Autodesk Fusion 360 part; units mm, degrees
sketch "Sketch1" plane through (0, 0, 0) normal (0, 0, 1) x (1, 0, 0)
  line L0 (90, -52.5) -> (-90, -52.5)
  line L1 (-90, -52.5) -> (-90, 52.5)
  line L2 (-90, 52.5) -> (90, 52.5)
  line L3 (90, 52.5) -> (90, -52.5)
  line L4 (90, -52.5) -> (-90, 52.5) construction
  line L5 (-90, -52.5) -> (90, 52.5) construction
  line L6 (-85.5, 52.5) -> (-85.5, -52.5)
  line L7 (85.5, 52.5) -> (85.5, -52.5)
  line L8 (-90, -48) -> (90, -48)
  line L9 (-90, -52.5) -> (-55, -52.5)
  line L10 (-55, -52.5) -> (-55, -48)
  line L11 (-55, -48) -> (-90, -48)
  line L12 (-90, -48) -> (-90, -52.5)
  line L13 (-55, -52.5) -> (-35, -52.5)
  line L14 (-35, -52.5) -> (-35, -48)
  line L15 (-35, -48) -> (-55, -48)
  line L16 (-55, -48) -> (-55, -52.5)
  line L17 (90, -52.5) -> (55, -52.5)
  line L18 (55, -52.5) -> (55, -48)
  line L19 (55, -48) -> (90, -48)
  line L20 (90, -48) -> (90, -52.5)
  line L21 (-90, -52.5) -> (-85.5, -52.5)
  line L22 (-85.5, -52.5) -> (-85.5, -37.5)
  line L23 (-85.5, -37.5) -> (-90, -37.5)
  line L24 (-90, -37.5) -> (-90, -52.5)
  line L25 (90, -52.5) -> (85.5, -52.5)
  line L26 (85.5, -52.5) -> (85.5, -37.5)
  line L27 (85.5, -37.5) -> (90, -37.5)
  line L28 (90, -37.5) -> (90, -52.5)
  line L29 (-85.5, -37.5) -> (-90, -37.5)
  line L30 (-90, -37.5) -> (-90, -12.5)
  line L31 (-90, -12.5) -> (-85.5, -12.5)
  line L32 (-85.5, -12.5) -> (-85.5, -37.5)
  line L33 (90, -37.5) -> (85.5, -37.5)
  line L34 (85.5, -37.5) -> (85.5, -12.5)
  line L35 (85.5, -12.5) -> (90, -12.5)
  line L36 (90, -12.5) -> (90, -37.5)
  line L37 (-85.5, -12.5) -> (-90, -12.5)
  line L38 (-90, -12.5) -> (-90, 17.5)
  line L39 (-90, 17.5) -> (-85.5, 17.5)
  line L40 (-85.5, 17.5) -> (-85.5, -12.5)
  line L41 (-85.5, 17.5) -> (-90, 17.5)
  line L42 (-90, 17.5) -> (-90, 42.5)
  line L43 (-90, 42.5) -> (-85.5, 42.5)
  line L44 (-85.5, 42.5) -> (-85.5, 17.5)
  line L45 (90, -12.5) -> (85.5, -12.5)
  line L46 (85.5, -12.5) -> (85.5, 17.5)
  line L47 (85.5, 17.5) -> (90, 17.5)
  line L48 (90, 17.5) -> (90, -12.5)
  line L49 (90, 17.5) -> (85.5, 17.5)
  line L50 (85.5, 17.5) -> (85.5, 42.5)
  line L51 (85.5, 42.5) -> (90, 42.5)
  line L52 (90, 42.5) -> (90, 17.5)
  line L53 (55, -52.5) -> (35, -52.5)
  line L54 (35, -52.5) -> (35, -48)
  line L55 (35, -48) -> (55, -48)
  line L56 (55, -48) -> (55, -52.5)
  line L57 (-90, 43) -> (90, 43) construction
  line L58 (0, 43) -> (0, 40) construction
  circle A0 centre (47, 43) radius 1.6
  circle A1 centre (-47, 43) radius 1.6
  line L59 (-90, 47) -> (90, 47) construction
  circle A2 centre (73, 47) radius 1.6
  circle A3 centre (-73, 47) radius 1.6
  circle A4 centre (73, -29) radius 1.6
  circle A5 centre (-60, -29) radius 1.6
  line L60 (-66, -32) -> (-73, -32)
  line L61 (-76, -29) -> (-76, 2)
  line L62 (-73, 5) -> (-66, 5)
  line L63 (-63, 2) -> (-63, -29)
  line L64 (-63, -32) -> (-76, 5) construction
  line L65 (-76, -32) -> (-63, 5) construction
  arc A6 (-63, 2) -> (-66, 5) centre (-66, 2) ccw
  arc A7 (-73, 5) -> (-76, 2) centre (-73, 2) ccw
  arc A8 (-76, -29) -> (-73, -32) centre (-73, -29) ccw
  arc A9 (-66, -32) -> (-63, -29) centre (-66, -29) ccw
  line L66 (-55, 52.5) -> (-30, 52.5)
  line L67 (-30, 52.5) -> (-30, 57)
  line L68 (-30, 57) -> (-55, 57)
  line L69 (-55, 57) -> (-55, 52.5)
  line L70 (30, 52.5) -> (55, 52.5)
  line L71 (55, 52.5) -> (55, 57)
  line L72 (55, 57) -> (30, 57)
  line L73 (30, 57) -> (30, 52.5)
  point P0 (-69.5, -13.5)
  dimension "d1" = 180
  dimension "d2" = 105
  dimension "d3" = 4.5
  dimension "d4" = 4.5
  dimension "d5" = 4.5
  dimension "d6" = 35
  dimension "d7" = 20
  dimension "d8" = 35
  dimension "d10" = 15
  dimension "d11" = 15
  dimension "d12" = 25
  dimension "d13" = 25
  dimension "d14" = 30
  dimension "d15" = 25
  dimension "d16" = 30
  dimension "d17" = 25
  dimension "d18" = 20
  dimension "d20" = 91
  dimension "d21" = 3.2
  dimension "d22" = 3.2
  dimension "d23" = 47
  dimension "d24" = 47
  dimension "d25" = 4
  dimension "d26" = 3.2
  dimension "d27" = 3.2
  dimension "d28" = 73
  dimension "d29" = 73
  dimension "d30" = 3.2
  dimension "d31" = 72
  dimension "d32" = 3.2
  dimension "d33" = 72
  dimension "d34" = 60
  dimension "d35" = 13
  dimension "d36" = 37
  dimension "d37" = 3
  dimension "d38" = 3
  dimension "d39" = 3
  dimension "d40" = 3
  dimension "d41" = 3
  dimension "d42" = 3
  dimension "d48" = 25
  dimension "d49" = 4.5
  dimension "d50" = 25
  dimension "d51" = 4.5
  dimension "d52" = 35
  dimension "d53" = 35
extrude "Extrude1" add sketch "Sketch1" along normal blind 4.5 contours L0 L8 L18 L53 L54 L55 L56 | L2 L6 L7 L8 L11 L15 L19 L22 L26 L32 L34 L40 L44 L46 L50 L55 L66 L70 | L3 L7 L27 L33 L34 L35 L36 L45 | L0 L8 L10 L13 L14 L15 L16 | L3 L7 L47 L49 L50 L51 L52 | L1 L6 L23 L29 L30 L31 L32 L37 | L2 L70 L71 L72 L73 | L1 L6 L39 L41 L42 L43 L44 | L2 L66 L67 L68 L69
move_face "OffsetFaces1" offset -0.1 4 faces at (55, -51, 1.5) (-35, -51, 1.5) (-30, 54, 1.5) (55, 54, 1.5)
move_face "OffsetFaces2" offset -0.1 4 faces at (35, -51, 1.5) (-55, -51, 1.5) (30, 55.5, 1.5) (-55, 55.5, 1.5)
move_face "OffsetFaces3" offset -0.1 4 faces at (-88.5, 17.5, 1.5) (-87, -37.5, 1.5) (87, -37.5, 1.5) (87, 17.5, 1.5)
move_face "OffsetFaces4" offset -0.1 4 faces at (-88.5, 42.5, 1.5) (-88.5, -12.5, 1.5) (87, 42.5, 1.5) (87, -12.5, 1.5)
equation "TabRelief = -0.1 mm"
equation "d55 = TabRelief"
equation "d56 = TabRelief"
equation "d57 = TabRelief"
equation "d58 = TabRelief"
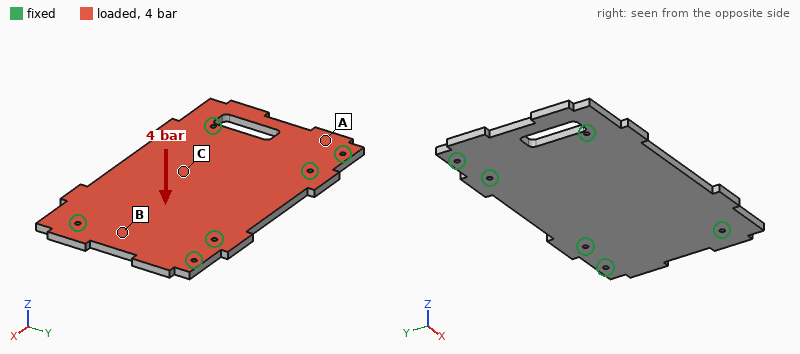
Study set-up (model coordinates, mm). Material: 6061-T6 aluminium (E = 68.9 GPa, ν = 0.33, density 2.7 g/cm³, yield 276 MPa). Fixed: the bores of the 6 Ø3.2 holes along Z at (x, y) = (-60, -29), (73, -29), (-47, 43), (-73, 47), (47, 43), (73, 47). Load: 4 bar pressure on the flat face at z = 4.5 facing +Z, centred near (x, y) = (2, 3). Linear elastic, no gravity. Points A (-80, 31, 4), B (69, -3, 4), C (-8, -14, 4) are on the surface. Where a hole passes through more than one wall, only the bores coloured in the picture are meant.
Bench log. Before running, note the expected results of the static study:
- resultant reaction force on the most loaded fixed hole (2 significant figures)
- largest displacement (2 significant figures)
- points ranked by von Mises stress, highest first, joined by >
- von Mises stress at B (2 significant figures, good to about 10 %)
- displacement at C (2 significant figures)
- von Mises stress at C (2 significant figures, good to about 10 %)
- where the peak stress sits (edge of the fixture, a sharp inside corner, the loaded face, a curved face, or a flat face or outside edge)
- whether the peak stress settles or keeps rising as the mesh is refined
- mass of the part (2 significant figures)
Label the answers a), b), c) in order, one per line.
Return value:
a) 1.8 kN
b) 0.83 mm
c) C > B > A
d) 50 MPa
e) 0.59 mm
f) 67 MPa
g) edge of the fixture
h) keeps rising
i) 210 g
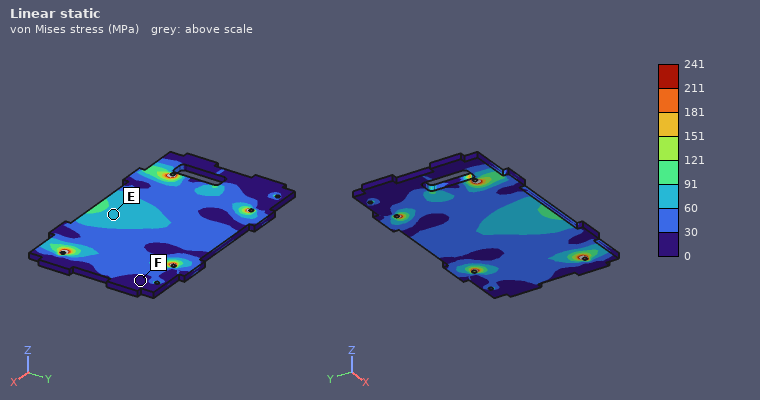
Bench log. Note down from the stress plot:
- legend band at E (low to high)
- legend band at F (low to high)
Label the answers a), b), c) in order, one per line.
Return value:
a) 60 to 91 MPa
b) 0 to 30 MPa
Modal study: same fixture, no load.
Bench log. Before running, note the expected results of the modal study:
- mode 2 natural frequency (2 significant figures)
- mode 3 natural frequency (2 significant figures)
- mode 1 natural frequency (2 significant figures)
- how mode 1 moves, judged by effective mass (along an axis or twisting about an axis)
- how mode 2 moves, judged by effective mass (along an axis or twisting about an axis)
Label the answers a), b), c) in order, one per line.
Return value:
a) 2300 Hz
b) 2500 Hz
c) 1300 Hz
d) along Z
e) along Z
